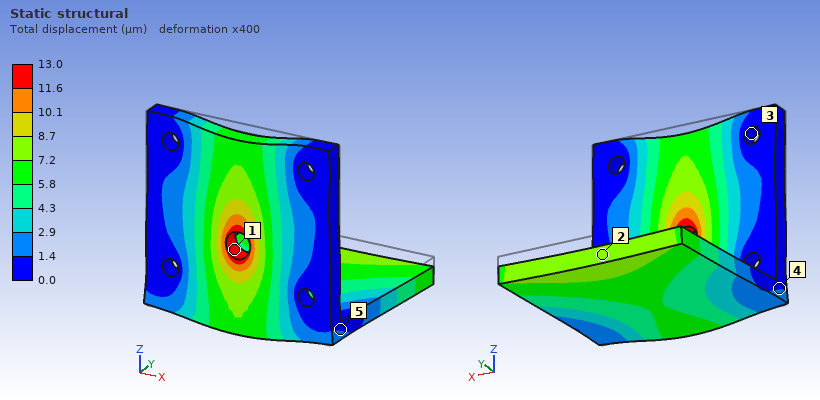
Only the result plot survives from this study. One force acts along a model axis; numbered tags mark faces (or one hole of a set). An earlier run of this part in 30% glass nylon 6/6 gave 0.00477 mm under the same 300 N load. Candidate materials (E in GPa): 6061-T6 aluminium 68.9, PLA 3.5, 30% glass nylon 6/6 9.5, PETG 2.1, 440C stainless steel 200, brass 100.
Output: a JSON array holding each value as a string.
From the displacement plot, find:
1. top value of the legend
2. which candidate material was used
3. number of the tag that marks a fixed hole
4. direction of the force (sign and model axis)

["13.0 µm", "PLA", "3", "-Z"]
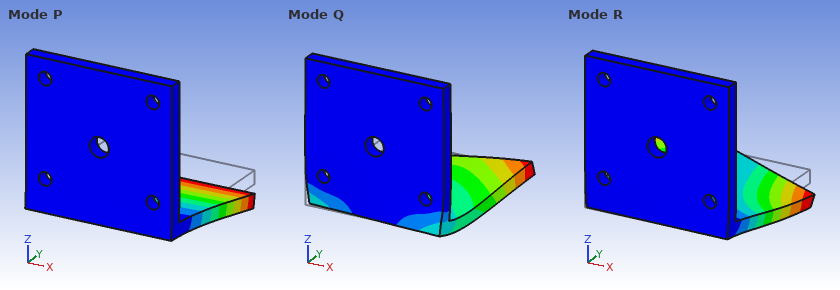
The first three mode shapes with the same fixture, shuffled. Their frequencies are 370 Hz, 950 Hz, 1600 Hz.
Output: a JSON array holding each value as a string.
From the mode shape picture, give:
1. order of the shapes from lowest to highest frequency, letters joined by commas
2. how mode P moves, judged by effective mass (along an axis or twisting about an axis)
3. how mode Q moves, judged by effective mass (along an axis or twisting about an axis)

["P, R, Q", "along Z", "along X"]
